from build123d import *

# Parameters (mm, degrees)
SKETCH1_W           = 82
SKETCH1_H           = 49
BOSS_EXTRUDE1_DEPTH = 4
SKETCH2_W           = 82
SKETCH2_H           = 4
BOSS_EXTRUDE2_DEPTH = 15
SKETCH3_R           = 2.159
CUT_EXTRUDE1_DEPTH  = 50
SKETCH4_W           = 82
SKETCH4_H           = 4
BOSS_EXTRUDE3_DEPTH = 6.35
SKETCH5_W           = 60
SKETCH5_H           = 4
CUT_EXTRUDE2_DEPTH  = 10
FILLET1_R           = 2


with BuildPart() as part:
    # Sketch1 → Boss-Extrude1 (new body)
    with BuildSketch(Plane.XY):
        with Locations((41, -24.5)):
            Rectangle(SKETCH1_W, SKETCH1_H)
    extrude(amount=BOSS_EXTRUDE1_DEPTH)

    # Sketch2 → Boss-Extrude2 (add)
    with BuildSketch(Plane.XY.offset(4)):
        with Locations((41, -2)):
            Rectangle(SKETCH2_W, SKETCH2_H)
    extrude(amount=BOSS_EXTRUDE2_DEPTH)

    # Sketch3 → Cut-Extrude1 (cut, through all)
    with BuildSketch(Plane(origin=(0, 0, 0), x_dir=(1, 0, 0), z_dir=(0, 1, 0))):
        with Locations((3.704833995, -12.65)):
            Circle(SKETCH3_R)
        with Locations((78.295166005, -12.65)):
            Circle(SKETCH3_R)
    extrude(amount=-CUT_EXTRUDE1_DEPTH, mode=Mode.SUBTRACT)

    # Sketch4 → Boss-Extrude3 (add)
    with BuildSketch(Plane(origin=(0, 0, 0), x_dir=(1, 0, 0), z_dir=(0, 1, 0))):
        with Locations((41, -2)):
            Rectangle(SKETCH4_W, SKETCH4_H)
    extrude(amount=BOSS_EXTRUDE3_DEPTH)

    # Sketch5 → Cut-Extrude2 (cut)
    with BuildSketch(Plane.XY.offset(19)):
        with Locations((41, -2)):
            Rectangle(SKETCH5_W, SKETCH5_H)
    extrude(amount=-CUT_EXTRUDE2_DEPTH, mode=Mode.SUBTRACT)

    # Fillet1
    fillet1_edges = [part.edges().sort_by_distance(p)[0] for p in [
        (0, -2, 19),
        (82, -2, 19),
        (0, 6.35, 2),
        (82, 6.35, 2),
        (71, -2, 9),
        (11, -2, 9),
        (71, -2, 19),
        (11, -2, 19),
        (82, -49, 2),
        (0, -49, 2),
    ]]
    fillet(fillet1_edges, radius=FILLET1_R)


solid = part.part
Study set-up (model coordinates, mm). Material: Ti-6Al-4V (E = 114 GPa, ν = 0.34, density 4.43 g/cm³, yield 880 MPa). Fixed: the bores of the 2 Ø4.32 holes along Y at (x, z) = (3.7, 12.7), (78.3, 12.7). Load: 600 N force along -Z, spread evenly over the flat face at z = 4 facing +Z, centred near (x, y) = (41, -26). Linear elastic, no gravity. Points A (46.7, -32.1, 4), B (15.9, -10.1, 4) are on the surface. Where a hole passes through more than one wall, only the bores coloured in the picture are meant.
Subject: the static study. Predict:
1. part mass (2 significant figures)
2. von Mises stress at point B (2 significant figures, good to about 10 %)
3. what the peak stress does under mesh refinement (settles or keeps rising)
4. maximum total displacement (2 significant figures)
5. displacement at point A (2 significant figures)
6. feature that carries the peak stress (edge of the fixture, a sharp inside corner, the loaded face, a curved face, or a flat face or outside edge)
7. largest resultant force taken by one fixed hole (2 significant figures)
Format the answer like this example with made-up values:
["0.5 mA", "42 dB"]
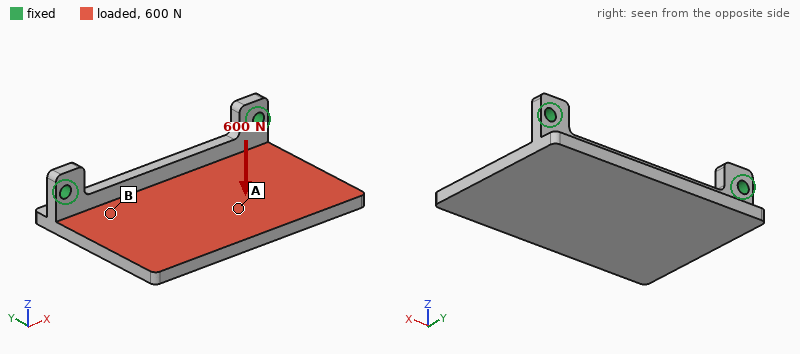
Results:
["91 g", "51 MPa", "keeps rising", "0.61 mm", "0.38 mm", "edge of the fixture", "420 N"]
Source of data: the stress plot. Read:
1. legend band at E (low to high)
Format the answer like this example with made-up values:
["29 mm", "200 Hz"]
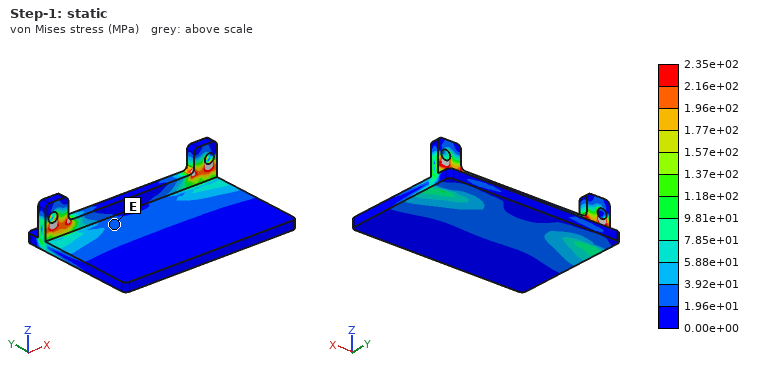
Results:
["1.96e+01 to 3.92e+01 MPa"]
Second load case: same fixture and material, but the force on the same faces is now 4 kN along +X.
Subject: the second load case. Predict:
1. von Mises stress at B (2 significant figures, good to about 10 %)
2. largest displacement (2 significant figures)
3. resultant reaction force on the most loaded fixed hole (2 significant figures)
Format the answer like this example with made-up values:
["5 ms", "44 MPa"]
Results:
["66 MPa", "0.19 mm", "2.4 kN"]
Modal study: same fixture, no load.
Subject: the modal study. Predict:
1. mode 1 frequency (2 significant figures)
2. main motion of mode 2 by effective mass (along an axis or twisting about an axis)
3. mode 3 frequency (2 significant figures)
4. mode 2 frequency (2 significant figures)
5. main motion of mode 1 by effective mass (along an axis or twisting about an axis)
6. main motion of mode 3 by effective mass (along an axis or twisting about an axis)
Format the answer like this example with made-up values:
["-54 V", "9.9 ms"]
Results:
["760 Hz", "twisting about Y", "4300 Hz", "2100 Hz", "along Z", "along Y"]
